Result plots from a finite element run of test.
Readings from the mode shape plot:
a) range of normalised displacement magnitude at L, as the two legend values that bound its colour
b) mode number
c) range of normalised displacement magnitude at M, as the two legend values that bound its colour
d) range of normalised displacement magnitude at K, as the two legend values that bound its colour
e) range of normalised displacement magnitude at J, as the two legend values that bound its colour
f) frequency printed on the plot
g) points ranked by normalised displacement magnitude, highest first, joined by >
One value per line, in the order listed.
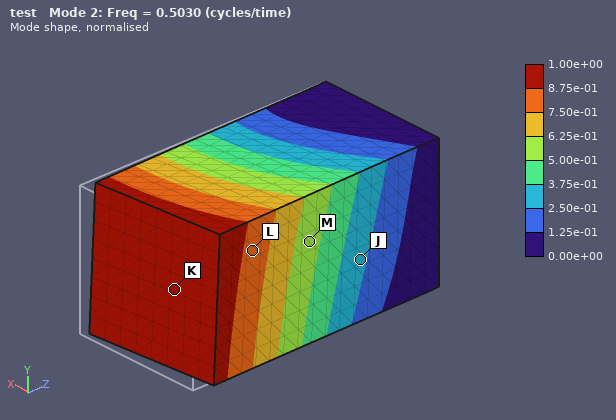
7.50e-01 to 8.75e-01
2
5.00e-01 to 6.25e-01
8.75e-01 to 1.00e+00
2.50e-01 to 3.75e-01
0.5030
K > L > M > J
